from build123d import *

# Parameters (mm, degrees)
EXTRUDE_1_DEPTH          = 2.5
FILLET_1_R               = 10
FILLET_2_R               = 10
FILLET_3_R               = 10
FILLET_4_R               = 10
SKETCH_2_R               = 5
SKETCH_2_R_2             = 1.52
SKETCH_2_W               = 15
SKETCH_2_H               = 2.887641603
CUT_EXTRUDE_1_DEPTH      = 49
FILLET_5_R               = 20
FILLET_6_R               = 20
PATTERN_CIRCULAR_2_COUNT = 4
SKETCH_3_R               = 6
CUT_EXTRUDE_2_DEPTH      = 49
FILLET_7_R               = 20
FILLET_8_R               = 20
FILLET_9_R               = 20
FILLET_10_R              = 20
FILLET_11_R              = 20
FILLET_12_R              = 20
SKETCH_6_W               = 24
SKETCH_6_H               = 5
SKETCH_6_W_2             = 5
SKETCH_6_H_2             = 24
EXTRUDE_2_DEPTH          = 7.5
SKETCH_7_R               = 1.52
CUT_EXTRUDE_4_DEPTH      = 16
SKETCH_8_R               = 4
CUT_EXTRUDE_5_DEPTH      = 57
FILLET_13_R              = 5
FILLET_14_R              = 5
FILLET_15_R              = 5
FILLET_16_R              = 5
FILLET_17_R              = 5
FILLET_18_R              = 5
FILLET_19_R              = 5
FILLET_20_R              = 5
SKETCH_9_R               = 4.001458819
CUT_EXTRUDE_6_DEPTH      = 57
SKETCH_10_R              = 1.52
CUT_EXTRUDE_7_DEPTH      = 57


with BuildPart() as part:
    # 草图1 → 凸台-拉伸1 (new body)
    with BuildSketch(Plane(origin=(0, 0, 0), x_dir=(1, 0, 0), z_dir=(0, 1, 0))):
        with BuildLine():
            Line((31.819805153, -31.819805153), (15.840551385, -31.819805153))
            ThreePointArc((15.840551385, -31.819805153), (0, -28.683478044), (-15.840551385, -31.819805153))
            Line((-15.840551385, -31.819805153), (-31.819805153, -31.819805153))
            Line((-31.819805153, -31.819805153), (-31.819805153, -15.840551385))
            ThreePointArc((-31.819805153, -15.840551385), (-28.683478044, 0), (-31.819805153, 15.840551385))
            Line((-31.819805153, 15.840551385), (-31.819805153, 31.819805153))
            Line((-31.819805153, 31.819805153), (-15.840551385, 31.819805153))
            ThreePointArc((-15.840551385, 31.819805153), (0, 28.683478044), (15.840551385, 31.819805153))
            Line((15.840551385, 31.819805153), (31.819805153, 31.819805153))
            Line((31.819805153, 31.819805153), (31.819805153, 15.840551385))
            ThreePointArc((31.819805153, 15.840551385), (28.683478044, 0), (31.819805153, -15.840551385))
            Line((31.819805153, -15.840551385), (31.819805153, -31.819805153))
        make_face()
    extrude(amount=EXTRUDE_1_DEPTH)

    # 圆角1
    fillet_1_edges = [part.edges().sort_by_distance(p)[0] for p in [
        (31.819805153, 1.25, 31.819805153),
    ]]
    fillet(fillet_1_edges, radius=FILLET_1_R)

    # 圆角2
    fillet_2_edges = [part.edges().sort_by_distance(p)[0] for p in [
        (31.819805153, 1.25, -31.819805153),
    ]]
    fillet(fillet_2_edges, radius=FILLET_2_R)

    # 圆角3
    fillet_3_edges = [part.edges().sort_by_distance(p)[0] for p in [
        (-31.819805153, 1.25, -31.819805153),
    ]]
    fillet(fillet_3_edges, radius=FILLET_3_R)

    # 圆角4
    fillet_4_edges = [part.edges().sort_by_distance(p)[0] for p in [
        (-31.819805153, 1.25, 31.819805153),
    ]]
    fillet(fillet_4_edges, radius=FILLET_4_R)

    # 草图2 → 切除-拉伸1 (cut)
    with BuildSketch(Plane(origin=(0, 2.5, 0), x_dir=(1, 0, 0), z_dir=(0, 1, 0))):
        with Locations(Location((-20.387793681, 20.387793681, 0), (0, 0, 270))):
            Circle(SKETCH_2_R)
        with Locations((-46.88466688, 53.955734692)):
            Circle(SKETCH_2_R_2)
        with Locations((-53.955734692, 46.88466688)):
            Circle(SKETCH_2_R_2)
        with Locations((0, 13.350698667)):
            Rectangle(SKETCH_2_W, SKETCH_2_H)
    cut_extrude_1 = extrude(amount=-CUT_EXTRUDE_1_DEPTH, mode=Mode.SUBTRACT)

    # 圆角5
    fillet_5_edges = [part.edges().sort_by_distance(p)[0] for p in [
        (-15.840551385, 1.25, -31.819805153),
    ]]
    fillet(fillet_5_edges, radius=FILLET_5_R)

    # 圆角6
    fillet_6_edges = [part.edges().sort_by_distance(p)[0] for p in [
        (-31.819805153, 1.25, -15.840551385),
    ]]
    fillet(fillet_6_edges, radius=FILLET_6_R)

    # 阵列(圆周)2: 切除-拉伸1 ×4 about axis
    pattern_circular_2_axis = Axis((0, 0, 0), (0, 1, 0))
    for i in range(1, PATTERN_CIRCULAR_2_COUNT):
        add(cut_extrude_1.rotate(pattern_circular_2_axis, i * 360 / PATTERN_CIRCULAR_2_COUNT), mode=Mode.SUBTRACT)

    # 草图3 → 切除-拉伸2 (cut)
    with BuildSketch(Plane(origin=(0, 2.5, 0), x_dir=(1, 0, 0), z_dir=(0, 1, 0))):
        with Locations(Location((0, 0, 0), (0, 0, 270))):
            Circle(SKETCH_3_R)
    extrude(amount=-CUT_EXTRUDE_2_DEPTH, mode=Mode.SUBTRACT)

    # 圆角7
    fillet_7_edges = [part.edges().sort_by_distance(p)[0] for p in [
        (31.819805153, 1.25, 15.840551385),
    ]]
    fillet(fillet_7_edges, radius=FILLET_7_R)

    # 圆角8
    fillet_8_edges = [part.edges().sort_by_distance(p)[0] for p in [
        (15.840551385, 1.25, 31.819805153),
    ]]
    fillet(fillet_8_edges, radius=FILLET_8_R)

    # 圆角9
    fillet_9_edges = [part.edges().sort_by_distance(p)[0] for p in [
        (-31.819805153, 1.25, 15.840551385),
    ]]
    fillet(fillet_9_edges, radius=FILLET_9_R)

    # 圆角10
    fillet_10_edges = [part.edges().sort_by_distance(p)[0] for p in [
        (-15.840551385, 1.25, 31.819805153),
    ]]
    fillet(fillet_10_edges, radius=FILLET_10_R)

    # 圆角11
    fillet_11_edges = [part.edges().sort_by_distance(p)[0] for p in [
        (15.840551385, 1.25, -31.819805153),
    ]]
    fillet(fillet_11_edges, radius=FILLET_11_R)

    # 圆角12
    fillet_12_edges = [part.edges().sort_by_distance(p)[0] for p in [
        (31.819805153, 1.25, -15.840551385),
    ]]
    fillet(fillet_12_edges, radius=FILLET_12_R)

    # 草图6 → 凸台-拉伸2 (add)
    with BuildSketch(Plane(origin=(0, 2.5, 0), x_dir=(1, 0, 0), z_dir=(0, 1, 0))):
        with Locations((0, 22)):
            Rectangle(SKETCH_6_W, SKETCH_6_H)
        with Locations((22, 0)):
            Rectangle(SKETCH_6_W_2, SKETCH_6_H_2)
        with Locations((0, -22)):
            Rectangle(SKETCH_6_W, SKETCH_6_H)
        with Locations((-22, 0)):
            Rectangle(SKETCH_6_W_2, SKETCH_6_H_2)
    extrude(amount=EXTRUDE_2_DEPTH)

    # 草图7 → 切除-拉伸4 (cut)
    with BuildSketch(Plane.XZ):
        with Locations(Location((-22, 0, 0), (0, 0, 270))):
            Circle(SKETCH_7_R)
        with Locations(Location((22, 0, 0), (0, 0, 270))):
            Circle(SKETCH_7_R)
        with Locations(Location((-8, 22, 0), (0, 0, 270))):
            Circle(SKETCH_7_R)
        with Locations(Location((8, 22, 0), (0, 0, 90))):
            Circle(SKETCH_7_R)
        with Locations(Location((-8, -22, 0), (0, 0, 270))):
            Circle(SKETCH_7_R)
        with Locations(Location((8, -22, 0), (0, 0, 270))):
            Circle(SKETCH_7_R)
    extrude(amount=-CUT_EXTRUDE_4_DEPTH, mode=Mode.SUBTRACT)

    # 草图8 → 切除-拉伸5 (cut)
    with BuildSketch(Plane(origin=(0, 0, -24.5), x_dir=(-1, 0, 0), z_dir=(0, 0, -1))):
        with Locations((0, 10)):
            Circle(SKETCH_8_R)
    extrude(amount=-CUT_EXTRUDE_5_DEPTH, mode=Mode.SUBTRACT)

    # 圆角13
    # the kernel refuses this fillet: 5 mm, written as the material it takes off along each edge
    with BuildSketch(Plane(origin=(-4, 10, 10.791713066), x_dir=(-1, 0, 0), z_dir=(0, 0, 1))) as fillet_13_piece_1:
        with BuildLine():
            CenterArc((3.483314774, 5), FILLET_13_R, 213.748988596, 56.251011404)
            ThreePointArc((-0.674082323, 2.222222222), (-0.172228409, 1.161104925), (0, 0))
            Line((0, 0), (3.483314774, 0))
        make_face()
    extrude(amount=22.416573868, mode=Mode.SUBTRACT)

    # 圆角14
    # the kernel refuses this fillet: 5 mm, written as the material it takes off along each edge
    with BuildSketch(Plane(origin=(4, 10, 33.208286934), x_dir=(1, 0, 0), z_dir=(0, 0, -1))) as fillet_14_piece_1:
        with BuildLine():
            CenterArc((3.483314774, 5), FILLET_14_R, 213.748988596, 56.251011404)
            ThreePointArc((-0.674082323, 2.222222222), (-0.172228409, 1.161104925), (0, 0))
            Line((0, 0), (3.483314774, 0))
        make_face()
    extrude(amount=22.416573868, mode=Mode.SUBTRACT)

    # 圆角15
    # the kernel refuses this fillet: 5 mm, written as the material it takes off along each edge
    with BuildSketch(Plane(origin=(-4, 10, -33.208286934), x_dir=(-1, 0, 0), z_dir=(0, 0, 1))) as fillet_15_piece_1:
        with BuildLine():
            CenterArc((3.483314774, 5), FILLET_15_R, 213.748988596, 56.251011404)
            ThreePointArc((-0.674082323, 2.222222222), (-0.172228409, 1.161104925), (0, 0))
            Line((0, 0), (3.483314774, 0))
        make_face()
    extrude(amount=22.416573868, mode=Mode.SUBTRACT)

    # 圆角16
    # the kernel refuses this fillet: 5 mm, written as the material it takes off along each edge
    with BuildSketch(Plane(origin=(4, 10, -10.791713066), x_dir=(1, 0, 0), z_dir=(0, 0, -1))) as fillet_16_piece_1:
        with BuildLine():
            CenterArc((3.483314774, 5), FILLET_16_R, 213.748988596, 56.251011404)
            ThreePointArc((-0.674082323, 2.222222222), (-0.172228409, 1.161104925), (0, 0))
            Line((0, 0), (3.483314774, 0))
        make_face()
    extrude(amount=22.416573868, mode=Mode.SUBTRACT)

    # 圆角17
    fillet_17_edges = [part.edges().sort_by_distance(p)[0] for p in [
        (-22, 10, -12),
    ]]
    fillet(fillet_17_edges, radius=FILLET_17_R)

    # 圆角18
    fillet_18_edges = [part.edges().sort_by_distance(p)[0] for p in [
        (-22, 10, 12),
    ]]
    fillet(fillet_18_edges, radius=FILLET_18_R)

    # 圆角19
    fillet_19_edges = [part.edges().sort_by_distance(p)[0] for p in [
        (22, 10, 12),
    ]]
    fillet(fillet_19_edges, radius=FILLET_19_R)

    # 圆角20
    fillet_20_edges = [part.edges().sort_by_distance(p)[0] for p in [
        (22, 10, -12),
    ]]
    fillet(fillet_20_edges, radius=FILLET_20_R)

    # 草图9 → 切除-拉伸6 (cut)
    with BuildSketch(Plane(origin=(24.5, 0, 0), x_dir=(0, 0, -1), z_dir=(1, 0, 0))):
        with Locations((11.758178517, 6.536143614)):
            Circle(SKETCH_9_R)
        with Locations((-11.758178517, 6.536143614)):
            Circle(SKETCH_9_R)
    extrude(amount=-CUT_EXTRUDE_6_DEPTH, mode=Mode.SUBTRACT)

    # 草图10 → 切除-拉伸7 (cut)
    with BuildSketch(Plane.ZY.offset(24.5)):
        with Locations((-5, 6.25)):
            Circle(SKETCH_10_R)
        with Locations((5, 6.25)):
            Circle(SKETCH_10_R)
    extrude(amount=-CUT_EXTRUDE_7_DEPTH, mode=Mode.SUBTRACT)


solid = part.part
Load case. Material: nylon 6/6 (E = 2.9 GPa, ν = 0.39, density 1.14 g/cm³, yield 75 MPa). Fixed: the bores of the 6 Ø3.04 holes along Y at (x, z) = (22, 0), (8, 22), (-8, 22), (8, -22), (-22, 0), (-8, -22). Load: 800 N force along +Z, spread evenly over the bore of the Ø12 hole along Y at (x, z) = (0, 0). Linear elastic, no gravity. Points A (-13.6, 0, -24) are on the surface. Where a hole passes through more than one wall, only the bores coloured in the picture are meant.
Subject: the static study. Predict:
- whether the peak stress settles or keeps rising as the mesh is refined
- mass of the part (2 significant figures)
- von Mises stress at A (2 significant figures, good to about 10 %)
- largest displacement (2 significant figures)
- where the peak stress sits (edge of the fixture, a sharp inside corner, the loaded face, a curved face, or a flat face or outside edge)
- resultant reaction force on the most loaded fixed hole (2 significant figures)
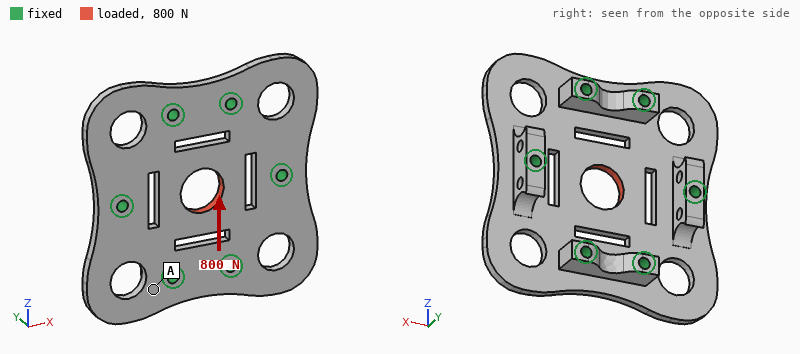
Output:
keeps rising
11 g
2.7 MPa
0.13 mm
a sharp inside corner
160 N
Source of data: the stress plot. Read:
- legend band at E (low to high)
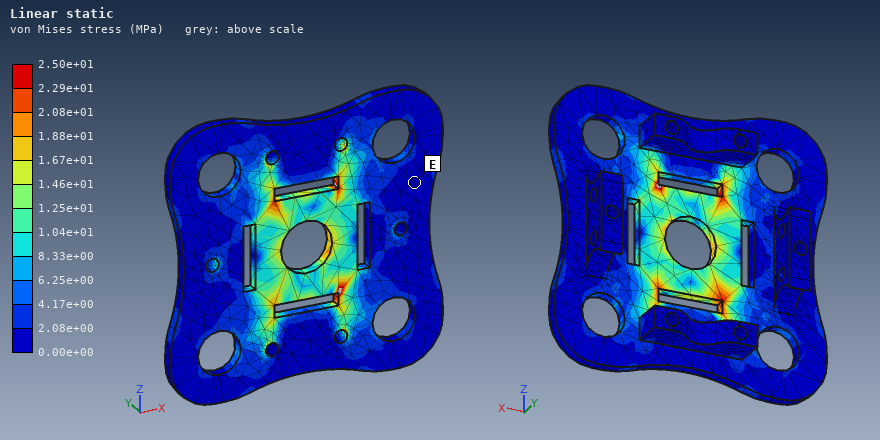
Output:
0.00e+00 to 2.08e+00 MPa
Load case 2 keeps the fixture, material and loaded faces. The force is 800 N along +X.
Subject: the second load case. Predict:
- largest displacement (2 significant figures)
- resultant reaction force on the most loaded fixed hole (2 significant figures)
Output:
0.14 mm
190 N
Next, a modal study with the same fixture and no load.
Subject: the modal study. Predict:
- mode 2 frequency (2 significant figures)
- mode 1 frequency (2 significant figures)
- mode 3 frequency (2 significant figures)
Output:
2200 Hz
2200 Hz
2200 Hz
